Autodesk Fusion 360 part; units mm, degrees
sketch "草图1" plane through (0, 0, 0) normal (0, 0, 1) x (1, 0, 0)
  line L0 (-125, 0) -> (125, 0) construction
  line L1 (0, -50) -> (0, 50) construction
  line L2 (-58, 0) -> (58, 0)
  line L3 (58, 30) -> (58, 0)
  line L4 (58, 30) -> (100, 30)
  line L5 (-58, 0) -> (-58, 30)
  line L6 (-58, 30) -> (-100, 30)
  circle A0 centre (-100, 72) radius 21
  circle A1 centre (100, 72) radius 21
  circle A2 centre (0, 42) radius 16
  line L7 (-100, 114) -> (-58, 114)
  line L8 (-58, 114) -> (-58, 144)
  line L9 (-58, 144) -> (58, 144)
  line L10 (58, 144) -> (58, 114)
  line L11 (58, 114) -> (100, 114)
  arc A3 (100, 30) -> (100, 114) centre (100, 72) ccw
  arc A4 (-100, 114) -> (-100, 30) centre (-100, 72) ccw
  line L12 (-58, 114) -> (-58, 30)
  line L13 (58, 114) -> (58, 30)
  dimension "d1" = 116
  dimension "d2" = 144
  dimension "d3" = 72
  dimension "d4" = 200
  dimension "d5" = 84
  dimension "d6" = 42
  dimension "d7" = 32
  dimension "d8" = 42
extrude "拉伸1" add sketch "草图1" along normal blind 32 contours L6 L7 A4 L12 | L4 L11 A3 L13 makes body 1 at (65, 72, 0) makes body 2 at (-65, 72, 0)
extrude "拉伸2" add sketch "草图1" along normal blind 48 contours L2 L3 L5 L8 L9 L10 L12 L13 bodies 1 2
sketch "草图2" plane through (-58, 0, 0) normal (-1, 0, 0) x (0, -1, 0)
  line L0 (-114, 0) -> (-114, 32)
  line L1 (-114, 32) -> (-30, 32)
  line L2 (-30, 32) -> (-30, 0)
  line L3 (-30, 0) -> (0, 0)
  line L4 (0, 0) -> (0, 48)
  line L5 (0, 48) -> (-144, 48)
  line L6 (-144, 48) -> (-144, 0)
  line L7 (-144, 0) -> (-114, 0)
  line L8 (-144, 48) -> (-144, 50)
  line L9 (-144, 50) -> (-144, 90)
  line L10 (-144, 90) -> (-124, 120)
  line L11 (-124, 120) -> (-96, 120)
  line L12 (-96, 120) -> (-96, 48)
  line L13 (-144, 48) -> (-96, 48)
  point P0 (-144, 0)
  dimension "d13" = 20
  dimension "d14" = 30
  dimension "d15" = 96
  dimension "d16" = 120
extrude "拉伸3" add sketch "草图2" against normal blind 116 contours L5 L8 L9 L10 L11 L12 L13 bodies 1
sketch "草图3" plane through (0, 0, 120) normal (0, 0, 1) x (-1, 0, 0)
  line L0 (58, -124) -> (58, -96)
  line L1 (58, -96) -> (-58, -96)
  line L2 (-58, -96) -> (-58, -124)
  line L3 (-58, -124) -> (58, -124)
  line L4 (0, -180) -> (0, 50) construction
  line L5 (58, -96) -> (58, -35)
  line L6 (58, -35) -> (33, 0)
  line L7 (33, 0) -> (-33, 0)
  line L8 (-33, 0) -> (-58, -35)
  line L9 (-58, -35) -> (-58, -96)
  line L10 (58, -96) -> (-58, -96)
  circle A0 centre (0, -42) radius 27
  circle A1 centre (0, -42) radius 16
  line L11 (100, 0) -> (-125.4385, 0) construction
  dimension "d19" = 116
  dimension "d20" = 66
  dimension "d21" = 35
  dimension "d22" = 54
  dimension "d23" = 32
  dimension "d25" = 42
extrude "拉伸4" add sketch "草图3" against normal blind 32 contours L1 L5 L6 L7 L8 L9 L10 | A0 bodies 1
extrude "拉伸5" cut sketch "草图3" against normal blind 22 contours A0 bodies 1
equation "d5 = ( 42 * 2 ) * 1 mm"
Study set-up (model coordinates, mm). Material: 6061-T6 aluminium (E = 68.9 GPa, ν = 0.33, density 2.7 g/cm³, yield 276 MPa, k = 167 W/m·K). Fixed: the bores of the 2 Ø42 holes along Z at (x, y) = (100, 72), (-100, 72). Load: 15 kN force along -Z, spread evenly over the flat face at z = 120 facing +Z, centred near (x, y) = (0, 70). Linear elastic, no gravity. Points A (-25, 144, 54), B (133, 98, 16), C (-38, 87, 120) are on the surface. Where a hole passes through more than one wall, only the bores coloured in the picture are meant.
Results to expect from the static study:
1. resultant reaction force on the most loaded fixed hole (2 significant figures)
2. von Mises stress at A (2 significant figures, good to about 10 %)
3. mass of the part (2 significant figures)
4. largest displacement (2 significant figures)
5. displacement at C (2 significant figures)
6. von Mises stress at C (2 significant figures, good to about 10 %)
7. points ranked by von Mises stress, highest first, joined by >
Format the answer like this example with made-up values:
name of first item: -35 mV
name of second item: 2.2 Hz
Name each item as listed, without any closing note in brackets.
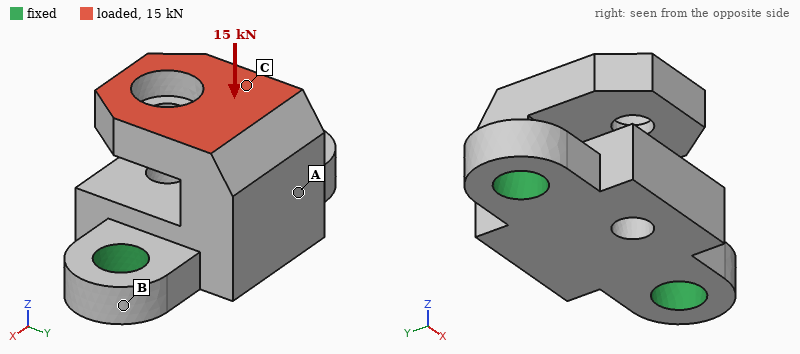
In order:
resultant reaction force on the most loaded fixed hole: 7.9 kN
von Mises stress at A: 12 MPa
mass of the part: 4.6 kg
largest displacement: 0.22 mm
displacement at C: 0.075 mm
von Mises stress at C: 19 MPa
points ranked by von Mises stress, highest first, joined by >: C > A > B
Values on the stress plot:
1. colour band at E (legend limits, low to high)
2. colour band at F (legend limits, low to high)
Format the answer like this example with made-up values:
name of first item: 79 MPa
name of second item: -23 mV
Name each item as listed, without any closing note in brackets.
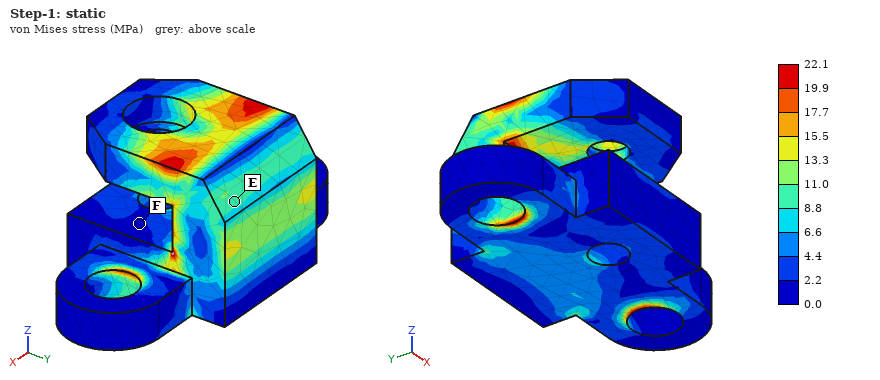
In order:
colour band at E: 8.8 to 11.0 MPa
colour band at F: 0.0 to 2.2 MPa
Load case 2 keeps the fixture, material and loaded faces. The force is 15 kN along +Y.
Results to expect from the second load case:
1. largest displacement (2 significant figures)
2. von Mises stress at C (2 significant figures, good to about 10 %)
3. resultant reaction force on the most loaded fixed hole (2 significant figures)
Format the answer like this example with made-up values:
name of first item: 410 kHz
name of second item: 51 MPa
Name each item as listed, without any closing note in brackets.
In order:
largest displacement: 0.37 mm
von Mises stress at C: 11 MPa
resultant reaction force on the most loaded fixed hole: 7.5 kN
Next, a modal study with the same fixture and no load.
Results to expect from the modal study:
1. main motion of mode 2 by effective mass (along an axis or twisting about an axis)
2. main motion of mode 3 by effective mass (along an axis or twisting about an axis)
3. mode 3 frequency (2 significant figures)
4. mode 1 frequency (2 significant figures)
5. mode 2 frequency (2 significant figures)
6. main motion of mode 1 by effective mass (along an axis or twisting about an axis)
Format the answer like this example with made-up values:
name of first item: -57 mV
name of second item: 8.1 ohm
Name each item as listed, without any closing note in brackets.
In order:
main motion of mode 2 by effective mass: along X
main motion of mode 3 by effective mass: along Z
mode 3 frequency: 1900 Hz
mode 1 frequency: 1100 Hz
mode 2 frequency: 1900 Hz
main motion of mode 1 by effective mass: along Y
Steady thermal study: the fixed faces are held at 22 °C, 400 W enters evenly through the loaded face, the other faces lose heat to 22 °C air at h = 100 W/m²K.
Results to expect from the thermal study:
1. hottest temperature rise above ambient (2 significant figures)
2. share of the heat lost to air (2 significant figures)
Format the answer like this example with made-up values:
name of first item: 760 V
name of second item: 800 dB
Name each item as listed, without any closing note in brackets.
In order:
hottest temperature rise above ambient: 52 K
share of the heat lost to air: 53 %
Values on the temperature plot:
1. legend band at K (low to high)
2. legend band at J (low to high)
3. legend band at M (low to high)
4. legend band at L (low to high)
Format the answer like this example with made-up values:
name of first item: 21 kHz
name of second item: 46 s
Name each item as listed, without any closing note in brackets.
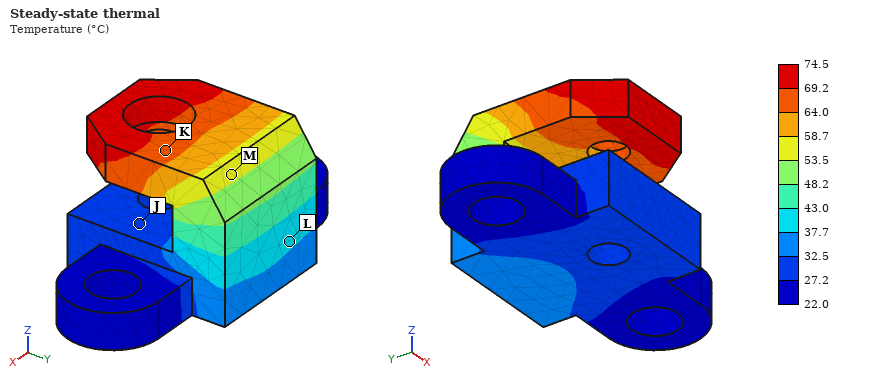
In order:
legend band at K: 64.0 to 69.2 °C
legend band at J: 27.2 to 32.5 °C
legend band at M: 53.5 to 58.7 °C
legend band at L: 37.7 to 43.0 °C
